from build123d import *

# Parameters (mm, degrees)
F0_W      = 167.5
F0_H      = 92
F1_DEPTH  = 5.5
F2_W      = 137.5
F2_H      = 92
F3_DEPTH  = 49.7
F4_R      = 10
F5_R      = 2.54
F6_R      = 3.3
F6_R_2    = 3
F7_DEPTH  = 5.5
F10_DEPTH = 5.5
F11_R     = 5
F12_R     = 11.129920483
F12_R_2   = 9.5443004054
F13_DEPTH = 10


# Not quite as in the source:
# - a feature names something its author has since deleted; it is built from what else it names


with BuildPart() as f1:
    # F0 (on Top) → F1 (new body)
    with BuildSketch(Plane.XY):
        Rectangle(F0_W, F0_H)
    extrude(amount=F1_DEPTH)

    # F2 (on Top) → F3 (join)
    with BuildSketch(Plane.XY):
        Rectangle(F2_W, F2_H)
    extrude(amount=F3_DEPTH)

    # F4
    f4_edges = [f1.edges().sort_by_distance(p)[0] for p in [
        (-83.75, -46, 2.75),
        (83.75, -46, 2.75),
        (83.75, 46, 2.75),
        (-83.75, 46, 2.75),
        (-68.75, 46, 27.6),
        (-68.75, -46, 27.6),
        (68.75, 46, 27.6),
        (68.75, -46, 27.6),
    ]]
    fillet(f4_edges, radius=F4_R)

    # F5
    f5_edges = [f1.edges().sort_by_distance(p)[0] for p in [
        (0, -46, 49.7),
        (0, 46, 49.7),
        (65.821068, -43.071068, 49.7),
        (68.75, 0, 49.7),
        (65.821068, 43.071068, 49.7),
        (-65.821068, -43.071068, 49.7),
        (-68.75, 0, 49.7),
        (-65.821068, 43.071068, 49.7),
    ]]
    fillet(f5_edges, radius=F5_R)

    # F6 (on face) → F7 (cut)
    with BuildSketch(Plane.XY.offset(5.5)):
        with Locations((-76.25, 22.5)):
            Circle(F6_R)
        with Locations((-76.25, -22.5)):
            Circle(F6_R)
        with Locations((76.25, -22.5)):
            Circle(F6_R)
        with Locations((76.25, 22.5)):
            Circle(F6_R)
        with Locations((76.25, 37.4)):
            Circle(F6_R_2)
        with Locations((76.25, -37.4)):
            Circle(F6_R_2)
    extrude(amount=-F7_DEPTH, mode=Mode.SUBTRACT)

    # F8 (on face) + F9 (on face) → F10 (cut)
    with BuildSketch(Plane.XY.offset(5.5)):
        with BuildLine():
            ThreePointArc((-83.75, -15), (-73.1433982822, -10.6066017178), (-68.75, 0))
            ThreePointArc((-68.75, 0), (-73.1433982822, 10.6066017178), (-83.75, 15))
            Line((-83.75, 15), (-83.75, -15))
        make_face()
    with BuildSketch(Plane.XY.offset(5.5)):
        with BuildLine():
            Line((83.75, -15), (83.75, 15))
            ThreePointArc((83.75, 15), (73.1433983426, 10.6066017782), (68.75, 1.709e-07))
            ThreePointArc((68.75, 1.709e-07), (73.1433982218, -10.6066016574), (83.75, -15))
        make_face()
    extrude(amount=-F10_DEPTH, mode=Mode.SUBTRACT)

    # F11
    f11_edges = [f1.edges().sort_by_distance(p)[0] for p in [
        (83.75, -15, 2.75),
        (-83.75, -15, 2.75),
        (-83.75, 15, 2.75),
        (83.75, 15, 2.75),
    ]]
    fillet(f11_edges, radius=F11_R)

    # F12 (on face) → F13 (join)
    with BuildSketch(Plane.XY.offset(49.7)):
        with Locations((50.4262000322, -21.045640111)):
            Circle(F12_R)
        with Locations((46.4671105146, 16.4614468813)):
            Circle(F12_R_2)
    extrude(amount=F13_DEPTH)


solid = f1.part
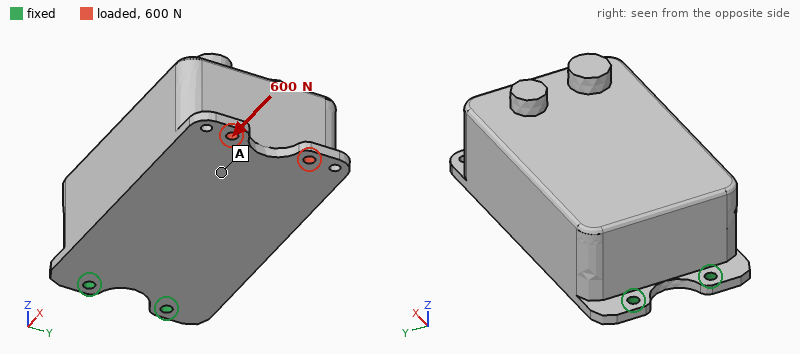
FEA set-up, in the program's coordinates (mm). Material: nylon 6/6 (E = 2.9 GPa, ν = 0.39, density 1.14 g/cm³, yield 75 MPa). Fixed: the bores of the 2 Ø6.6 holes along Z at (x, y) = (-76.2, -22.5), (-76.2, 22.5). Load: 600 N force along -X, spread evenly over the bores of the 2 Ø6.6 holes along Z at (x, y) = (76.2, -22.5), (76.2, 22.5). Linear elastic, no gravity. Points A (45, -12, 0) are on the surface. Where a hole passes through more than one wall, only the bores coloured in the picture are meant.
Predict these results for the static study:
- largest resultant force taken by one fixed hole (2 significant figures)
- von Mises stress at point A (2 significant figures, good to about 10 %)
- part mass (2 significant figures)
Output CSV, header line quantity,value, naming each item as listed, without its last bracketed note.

quantity,value
largest resultant force taken by one fixed hole,300 N
von Mises stress at point A,0.64 MPa
part mass,730 g
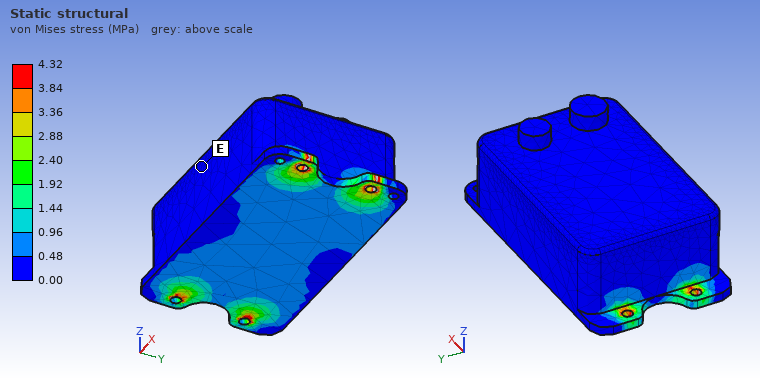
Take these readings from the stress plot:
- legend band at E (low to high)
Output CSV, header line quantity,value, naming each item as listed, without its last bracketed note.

quantity,value
legend band at E,0.00 to 0.48 MPa
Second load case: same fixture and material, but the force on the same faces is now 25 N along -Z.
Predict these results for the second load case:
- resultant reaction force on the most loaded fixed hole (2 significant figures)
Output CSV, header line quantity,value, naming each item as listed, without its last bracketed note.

quantity,value
resultant reaction force on the most loaded fixed hole,13 N
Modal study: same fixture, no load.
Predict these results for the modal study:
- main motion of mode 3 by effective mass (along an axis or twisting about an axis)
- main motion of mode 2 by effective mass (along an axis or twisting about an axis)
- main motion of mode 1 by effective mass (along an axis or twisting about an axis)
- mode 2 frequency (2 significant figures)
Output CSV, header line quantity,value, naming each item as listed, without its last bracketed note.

quantity,value
main motion of mode 3 by effective mass,twisting about X
main motion of mode 2 by effective mass,along Y
main motion of mode 1 by effective mass,along Z
mode 2 frequency,270 Hz
